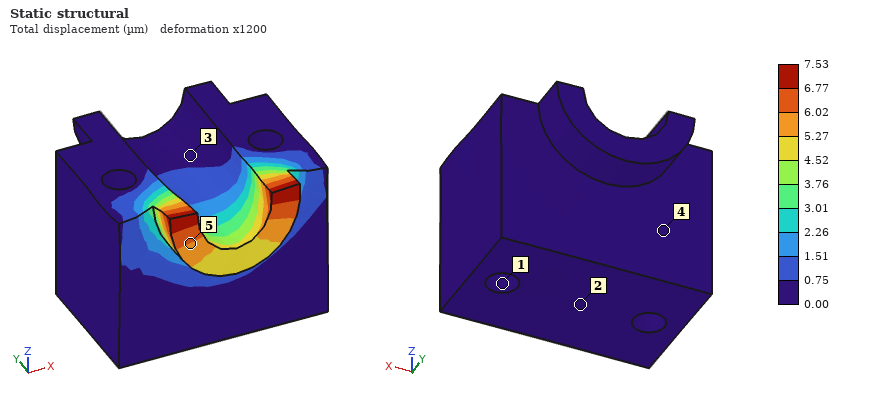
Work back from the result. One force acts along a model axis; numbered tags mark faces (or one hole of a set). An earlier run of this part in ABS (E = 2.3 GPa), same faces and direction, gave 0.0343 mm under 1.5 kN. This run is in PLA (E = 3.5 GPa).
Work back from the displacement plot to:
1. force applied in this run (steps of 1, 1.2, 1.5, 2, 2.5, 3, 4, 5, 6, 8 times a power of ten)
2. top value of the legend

500 N
7.53 µm
